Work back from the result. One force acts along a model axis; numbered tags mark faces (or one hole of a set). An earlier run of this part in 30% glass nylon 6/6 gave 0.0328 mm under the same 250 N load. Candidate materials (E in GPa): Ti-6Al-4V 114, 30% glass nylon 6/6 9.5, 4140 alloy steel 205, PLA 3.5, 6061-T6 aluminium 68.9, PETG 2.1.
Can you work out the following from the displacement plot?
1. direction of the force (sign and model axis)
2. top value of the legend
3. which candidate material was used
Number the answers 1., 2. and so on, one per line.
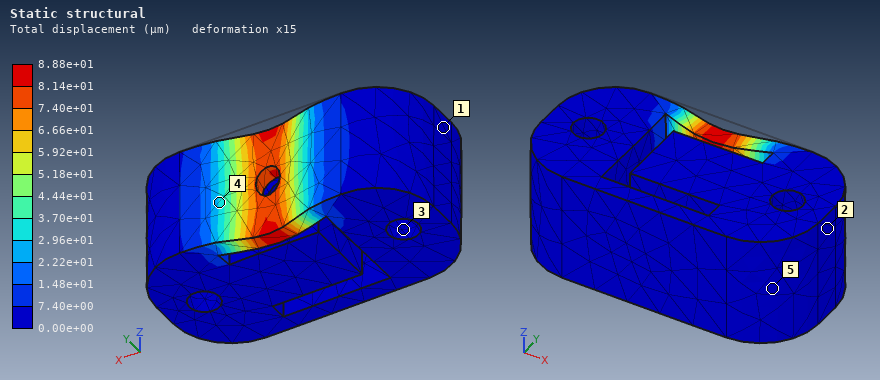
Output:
1. -Y
2. 8.88e+01 µm
3. PLA
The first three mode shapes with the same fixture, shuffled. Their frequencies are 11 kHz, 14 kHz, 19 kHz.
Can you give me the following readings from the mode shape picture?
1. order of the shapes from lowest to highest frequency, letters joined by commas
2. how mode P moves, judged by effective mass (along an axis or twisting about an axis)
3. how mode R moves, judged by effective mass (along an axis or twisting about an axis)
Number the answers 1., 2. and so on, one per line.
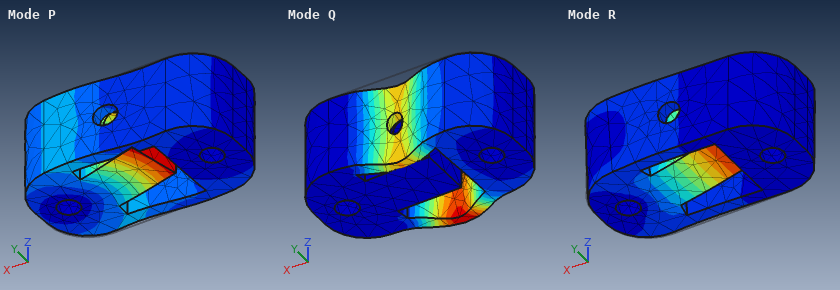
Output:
1. P, R, Q
2. along Y
3. along Z
